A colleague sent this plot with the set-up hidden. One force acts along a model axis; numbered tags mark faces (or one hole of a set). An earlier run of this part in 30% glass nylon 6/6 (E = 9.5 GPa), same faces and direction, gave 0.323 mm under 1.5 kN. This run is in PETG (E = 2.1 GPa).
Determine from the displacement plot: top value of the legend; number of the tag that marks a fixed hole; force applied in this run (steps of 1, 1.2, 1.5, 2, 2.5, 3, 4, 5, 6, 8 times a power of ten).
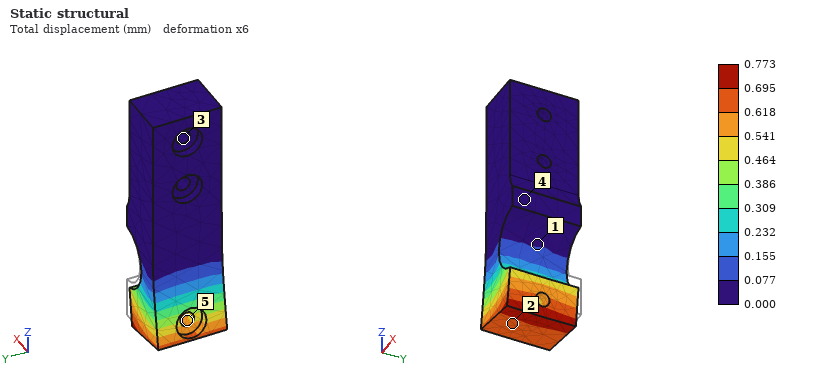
0.773 mm
3
800 N
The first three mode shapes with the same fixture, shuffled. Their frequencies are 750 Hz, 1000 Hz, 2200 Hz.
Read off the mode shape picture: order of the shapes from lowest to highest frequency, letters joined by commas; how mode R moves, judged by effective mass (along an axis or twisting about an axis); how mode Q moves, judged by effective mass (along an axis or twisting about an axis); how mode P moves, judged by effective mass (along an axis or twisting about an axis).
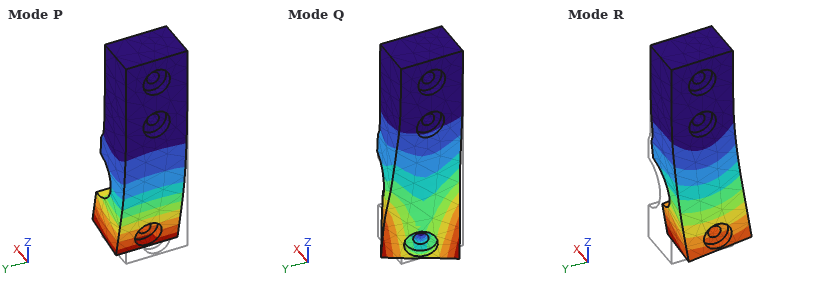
P, R, Q
along Y
twisting about Z
along X
